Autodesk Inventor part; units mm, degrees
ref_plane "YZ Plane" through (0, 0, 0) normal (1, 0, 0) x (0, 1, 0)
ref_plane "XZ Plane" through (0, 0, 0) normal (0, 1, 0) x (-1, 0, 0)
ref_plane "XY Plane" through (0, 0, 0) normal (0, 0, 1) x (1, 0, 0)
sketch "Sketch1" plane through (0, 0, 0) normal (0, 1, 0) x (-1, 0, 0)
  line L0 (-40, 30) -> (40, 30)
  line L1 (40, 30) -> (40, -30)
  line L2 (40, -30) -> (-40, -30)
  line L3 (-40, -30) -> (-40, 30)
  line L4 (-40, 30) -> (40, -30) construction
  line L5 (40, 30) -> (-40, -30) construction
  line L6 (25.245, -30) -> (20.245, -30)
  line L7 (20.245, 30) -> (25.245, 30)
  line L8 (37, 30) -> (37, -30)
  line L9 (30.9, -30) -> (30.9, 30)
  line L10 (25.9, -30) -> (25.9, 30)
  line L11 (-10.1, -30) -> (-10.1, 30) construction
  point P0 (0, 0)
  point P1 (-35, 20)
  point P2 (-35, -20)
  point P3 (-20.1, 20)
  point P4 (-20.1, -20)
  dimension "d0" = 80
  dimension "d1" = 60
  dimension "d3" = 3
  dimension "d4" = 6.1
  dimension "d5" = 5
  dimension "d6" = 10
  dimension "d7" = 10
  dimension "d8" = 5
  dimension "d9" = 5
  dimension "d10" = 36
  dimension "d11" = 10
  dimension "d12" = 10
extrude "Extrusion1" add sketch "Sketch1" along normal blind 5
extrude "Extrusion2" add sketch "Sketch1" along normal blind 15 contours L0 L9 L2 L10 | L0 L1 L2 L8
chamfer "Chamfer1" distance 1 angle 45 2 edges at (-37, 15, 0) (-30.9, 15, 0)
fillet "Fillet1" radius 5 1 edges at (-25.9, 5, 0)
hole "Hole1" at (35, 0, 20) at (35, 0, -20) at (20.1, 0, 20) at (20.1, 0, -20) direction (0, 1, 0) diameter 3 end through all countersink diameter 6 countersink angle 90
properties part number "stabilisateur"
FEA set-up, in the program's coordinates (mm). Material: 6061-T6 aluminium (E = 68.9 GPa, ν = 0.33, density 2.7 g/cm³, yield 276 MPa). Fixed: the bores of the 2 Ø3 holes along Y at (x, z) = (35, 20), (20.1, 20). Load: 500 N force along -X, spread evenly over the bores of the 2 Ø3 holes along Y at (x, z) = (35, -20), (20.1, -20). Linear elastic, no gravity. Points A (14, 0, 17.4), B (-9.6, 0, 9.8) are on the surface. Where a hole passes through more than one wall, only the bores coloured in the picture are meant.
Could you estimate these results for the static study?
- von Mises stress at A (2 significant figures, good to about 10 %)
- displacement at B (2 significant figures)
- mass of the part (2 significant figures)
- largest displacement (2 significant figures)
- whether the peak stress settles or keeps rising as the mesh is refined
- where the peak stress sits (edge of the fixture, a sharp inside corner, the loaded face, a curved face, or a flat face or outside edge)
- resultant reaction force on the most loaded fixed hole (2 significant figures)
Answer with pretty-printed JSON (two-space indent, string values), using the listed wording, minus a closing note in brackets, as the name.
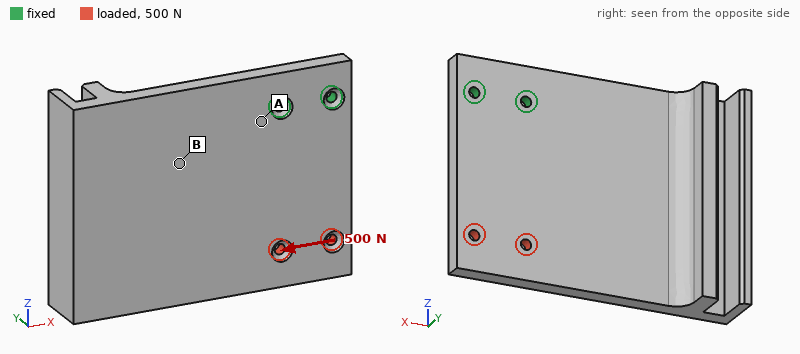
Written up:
{
  "von Mises stress at A": "8.5 MPa",
  "displacement at B": "22 µm",
  "mass of the part": "78 g",
  "largest displacement": "54 µm",
  "whether the peak stress settles or keeps rising as the mesh is refined": "keeps rising",
  "where the peak stress sits": "edge of the fixture",
  "resultant reaction force on the most loaded fixed hole": "1.2 kN"
}
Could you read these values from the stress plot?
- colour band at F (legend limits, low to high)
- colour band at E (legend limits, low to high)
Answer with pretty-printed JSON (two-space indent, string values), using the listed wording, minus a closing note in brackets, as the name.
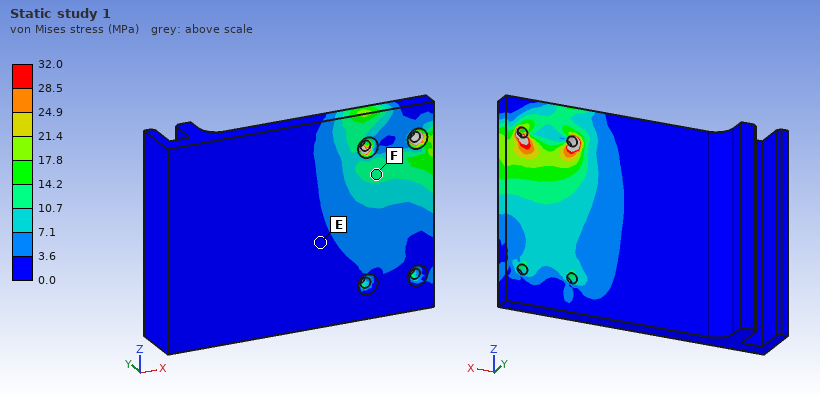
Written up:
{
  "colour band at F": "10.7 to 14.2 MPa",
  "colour band at E": "0.0 to 3.6 MPa"
}
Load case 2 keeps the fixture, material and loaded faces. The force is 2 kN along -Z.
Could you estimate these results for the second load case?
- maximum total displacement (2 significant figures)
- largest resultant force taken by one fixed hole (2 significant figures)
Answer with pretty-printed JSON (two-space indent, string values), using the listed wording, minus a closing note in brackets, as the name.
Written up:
{
  "maximum total displacement": "59 µm",
  "largest resultant force taken by one fixed hole": "1.0 kN"
}
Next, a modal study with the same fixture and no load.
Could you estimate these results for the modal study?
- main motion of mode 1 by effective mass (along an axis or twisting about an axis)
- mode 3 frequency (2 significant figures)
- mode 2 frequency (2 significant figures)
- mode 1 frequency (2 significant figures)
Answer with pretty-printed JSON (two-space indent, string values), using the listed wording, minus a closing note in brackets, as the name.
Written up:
{
  "main motion of mode 1 by effective mass": "along Y",
  "mode 3 frequency": "2100 Hz",
  "mode 2 frequency": "1100 Hz",
  "mode 1 frequency": "560 Hz"
}
